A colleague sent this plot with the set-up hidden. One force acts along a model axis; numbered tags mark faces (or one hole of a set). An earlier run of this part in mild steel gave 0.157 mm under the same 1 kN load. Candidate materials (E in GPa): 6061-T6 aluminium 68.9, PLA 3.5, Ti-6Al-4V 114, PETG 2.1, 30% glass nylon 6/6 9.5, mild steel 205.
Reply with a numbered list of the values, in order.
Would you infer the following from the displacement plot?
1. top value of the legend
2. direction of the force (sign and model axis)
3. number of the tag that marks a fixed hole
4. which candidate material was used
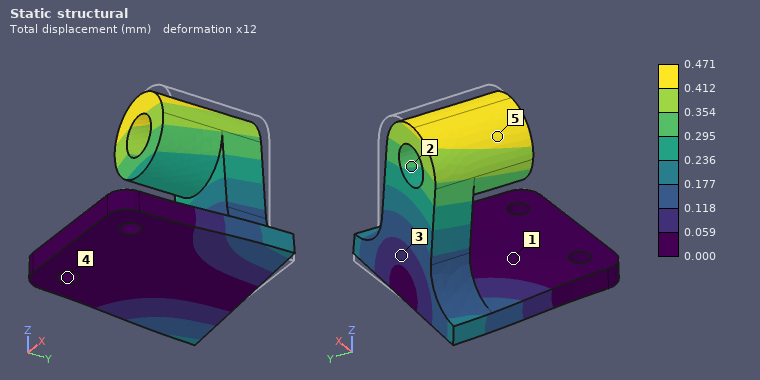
1. 0.471 mm
2. -X
3. 4
4. 6061-T6 aluminium
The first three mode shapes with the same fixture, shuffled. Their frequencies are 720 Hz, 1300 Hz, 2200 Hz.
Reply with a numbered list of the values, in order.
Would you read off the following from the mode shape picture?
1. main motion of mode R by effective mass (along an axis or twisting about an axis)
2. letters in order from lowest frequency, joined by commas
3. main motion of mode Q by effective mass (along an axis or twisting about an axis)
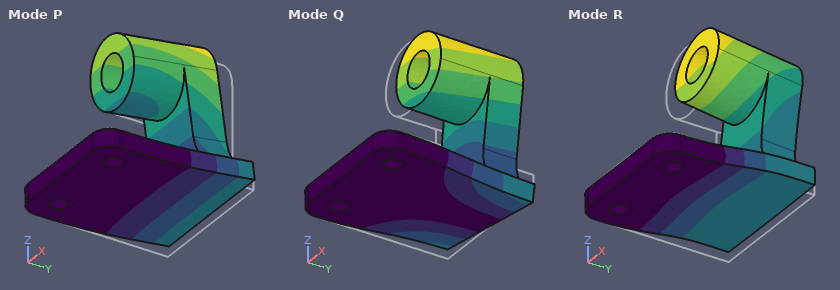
1. along Z
2. P, Q, R
3. along X
